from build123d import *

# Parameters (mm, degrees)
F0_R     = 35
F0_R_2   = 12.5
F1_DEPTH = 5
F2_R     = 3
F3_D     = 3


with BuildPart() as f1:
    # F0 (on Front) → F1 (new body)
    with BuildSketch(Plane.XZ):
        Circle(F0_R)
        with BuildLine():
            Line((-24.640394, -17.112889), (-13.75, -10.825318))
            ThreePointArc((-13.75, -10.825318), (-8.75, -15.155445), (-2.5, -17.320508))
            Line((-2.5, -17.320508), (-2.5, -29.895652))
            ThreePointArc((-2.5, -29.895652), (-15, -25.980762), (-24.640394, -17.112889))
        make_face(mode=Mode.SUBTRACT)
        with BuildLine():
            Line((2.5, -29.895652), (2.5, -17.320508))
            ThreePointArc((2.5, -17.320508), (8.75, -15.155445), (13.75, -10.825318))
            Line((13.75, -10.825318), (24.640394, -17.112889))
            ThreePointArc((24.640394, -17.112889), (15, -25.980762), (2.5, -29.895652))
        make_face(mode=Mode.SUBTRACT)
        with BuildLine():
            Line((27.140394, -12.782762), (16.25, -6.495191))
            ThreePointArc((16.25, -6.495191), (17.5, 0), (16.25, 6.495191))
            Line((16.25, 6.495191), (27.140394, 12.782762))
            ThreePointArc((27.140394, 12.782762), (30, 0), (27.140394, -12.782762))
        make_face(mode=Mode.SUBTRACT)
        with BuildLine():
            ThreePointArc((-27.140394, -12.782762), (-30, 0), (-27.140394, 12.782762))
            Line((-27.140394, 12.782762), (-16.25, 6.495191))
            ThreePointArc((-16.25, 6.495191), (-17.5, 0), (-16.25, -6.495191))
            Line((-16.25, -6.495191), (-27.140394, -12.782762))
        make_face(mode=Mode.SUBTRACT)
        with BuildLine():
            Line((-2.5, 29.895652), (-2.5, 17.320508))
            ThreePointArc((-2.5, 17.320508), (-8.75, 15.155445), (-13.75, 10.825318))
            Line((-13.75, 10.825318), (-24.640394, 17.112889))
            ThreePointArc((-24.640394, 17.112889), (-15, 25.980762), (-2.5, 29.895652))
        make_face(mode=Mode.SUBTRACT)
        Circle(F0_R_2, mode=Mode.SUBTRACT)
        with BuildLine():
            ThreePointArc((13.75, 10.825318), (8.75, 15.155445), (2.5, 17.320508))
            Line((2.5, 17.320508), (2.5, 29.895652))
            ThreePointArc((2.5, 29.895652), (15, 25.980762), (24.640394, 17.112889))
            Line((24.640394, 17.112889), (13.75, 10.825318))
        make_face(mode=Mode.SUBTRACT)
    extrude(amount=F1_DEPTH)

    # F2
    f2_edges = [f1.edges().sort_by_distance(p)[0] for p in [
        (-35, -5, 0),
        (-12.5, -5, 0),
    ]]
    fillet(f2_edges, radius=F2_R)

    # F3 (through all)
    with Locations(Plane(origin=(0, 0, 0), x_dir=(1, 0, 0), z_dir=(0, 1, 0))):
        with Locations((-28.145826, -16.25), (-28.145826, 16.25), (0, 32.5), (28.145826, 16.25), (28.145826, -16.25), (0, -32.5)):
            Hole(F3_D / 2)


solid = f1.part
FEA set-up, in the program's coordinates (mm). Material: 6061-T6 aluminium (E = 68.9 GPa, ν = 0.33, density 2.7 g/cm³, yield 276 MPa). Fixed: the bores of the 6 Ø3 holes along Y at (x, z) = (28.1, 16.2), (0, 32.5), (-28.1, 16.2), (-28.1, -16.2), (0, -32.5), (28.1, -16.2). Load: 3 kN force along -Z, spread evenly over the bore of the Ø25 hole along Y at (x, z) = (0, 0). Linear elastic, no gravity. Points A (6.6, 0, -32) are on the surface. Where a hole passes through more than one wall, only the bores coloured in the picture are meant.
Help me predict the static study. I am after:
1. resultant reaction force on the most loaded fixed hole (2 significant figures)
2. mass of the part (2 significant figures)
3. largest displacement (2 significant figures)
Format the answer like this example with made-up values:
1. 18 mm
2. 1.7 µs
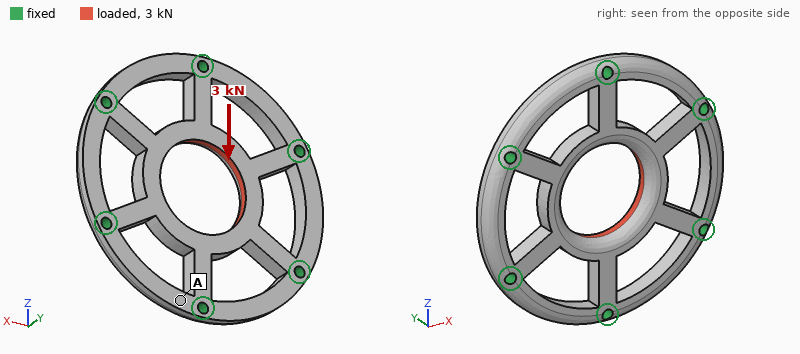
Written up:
1. 900 N
2. 23 g
3. 16 µm
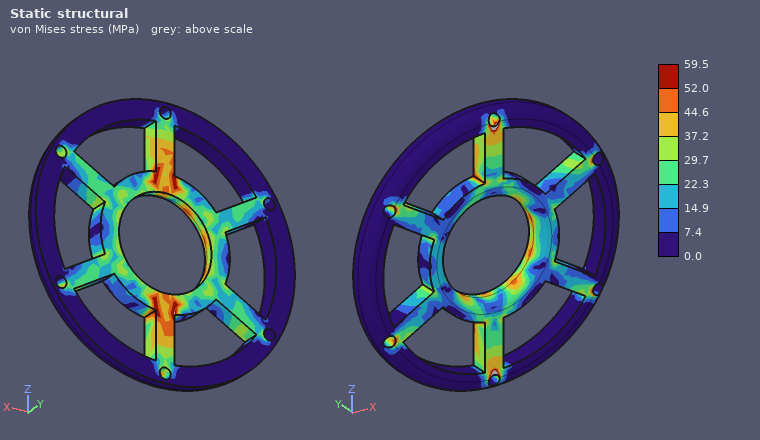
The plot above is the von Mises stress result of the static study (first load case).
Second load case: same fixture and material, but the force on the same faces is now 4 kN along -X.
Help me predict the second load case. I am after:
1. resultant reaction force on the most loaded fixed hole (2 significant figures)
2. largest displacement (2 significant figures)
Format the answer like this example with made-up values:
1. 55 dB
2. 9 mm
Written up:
1. 1.0 kN
2. 22 µm
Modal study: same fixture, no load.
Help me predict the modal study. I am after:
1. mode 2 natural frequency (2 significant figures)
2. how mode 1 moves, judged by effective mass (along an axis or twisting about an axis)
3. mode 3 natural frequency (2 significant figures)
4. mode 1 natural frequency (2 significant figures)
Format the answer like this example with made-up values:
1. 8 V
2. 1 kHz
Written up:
1. 13 kHz
2. along Y
3. 13 kHz
4. 8900 Hz
